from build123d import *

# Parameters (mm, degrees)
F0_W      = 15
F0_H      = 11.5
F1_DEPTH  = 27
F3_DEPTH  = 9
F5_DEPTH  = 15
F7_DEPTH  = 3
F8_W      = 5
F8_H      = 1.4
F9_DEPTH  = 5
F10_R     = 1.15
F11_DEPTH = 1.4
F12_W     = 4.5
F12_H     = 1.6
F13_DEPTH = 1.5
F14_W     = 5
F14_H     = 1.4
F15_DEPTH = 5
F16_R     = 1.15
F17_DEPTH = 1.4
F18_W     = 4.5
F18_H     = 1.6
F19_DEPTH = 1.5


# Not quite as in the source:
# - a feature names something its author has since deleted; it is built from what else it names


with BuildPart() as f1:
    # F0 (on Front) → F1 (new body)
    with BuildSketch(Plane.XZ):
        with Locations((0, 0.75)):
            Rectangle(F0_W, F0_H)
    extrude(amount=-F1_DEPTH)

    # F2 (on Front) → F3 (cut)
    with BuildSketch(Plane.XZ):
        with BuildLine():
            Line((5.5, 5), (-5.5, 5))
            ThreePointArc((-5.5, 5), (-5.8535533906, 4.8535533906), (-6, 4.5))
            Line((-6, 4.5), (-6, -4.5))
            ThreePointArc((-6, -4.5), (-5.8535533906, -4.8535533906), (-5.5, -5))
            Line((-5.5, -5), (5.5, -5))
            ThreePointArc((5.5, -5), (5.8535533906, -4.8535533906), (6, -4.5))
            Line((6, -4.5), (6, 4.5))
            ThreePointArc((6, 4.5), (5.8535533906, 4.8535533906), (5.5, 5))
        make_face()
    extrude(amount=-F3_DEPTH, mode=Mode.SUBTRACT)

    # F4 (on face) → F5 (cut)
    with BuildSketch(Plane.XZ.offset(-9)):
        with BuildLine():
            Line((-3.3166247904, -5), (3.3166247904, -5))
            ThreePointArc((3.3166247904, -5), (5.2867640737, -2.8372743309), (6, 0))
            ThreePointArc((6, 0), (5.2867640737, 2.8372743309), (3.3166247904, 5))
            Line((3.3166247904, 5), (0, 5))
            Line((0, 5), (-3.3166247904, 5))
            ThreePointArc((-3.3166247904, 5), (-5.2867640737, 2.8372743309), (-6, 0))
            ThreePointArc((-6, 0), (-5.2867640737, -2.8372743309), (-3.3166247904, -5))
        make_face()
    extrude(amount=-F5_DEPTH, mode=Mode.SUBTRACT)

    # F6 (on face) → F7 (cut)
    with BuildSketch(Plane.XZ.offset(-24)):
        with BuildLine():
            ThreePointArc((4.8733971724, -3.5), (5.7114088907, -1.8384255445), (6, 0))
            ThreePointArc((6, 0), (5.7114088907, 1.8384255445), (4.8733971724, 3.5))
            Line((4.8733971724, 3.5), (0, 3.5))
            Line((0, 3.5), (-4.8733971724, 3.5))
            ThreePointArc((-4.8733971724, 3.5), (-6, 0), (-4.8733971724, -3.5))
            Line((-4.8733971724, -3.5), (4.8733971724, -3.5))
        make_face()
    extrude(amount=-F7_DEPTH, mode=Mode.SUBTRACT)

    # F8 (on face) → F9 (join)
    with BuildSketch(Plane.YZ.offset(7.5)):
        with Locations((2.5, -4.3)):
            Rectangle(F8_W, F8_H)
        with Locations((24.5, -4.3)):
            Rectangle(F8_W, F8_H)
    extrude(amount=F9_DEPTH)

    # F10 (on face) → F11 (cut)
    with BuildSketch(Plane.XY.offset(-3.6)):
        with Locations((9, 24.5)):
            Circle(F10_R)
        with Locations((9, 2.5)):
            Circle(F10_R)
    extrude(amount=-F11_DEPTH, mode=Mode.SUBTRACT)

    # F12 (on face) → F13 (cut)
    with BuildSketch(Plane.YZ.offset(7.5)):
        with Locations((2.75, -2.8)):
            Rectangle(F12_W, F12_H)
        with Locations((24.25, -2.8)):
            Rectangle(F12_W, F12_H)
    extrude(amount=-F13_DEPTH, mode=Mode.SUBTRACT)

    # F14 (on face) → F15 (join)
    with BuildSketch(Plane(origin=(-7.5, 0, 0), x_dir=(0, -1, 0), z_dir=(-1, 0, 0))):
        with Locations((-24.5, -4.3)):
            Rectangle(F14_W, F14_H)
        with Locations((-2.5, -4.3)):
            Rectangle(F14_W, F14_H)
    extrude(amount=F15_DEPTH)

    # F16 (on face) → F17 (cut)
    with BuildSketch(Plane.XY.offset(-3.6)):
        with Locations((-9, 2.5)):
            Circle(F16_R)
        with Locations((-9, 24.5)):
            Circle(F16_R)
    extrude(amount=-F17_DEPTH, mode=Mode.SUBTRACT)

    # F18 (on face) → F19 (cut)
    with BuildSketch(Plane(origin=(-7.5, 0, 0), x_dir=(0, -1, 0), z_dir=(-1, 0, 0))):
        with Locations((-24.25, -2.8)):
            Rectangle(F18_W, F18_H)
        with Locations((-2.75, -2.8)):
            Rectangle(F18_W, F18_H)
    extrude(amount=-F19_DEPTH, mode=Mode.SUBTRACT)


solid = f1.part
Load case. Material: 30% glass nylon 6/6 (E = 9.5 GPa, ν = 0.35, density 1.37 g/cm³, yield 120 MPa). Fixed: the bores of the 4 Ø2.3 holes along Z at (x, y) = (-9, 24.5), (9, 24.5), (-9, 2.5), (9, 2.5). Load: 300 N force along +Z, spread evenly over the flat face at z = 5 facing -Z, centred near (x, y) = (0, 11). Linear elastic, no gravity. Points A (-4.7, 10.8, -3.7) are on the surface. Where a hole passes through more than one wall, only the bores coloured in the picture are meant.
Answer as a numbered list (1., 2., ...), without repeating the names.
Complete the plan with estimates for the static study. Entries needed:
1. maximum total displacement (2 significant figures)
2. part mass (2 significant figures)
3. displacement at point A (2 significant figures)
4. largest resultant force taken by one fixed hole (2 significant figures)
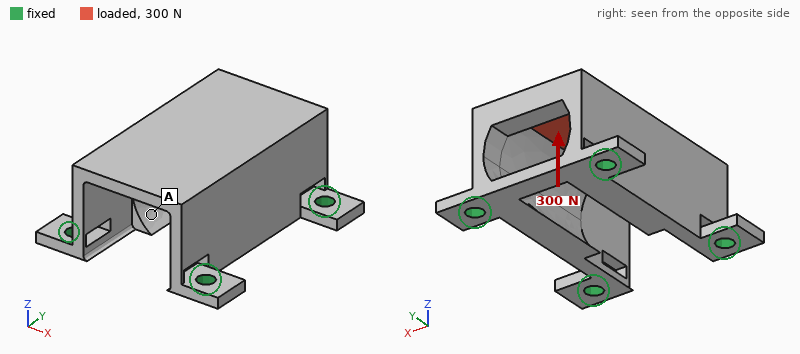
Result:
1. 0.14 mm
2. 2.5 g
3. 0.038 mm
4. 100 N
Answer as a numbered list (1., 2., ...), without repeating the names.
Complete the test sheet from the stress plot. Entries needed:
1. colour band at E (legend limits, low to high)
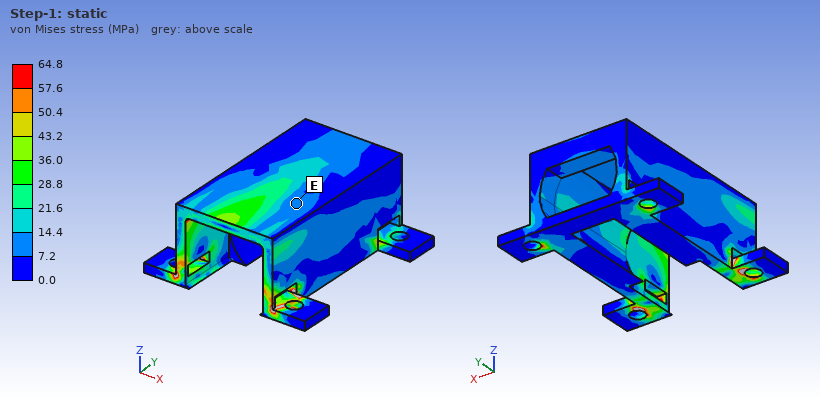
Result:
1. 7.2 to 14.4 MPa
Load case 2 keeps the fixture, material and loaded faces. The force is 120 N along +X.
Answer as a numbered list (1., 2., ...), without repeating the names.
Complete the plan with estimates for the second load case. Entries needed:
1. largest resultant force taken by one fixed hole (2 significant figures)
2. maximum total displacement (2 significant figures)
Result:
1. 84 N
2. 0.16 mm
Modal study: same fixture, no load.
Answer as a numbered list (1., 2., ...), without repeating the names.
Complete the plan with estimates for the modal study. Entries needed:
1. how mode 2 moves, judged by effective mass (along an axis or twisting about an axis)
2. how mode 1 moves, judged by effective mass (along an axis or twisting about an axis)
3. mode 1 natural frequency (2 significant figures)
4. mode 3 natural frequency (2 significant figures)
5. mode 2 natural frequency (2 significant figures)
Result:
1. twisting about Z
2. along X
3. 4200 Hz
4. 9200 Hz
5. 8600 Hz
